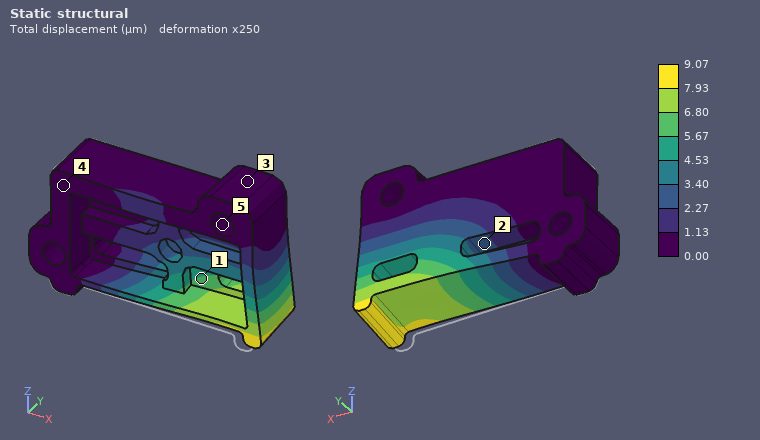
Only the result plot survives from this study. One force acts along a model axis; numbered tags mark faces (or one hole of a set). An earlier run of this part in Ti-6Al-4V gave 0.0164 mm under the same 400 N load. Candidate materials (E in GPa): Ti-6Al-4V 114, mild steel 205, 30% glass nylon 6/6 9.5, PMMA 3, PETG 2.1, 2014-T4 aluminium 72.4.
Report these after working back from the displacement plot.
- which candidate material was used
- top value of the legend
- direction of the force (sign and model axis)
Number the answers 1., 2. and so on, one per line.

1. mild steel
2. 9.07 µm
3. +Y
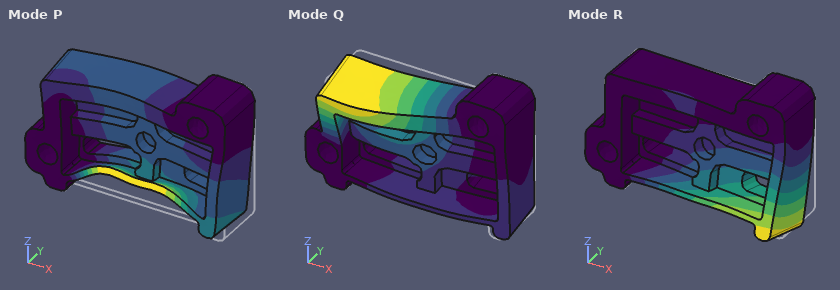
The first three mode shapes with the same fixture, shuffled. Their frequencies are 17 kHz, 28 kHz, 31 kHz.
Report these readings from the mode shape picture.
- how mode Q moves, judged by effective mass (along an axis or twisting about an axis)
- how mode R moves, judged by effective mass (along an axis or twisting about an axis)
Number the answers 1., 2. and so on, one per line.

1. along Y
2. along Y
